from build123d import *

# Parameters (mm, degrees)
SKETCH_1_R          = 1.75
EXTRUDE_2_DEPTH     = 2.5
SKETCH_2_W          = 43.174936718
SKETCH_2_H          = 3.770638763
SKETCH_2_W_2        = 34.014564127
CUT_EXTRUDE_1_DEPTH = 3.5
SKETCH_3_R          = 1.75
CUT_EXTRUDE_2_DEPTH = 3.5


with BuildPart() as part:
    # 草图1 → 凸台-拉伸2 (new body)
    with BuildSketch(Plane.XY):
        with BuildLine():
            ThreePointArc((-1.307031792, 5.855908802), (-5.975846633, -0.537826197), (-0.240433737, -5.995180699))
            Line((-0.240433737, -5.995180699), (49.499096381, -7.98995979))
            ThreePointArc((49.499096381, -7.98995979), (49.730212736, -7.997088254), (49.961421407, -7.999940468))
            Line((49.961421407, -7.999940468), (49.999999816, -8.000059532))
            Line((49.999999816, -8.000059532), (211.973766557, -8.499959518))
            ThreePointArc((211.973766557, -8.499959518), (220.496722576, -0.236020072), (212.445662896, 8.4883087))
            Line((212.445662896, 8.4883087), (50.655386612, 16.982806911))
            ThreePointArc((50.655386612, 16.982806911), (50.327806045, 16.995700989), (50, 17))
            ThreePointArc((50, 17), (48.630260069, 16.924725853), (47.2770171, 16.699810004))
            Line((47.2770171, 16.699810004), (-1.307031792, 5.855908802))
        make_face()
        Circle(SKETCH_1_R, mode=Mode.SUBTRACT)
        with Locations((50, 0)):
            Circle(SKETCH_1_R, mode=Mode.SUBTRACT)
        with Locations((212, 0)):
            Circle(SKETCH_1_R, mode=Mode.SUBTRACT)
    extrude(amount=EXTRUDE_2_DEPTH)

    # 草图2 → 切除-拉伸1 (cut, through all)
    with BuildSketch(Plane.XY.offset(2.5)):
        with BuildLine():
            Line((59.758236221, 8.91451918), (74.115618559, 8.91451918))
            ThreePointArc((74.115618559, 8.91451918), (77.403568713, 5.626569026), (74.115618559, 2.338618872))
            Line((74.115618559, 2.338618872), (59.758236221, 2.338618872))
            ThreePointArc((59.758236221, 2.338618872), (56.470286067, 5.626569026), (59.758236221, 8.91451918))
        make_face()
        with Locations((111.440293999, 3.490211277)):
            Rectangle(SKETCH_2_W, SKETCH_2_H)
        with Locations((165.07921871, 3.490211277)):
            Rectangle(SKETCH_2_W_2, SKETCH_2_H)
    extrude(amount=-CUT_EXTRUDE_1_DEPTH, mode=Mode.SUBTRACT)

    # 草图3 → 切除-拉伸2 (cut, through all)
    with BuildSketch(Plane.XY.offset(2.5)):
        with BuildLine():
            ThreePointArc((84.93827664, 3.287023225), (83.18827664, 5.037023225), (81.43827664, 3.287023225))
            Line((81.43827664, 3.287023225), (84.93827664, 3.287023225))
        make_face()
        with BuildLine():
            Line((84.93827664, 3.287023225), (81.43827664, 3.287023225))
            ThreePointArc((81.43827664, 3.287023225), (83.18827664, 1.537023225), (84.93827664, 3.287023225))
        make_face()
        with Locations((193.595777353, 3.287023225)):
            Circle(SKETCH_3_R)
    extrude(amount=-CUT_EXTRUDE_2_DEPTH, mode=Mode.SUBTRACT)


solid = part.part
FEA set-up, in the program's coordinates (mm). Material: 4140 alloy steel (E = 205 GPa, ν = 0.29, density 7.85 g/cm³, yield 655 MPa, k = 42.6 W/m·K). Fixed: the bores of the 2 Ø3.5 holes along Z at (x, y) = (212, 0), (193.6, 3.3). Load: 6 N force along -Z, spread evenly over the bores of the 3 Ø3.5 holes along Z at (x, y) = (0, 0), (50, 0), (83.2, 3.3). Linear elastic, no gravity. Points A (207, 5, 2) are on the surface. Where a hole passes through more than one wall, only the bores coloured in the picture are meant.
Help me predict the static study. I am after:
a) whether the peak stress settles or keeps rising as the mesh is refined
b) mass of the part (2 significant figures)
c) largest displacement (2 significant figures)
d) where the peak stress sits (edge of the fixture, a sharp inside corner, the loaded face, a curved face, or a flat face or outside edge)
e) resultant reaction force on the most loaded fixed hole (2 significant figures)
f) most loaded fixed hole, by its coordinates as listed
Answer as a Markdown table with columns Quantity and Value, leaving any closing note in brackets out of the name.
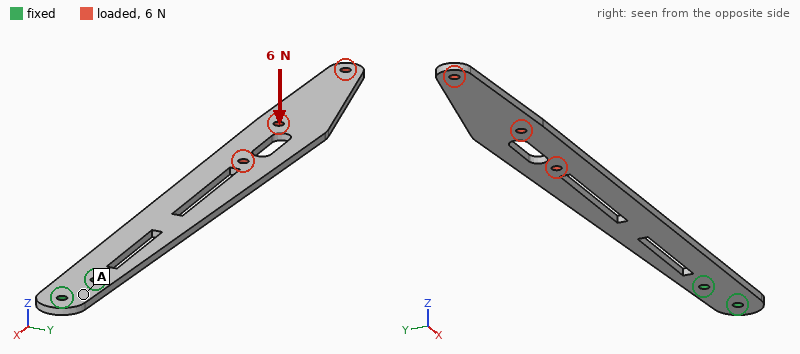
| Quantity | Value |
|---|---|
| whether the peak stress settles or keeps rising as the mesh is refined | keeps rising |
| mass of the part | 79 g |
| largest displacement | 2.2 mm |
| where the peak stress sits | edge of the fixture |
| resultant reaction force on the most loaded fixed hole | 18 N |
| most loaded fixed hole, by its coordinates as listed | (193.6, 3.3) |
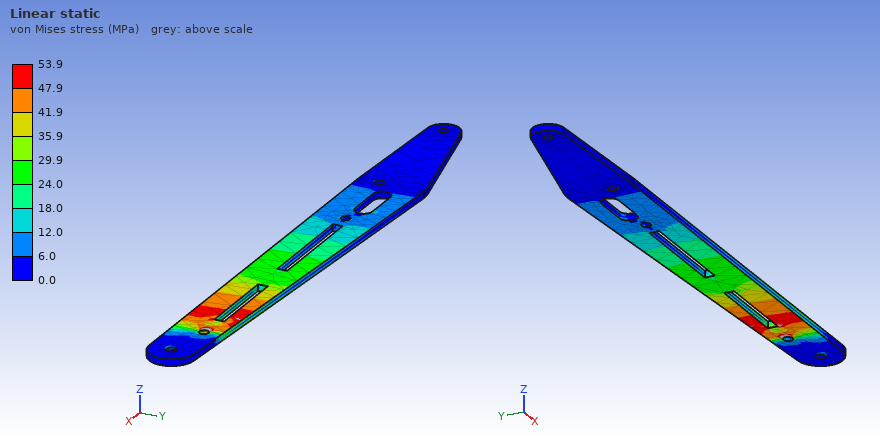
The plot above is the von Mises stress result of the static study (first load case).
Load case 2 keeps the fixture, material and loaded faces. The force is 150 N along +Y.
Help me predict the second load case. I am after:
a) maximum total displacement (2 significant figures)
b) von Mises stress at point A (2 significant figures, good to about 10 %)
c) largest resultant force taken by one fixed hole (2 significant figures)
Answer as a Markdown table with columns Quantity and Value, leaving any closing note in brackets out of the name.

| Quantity | Value |
|---|---|
| maximum total displacement | 0.99 mm |
| von Mises stress at point A | 29 MPa |
| largest resultant force taken by one fixed hole | 1.2 kN |
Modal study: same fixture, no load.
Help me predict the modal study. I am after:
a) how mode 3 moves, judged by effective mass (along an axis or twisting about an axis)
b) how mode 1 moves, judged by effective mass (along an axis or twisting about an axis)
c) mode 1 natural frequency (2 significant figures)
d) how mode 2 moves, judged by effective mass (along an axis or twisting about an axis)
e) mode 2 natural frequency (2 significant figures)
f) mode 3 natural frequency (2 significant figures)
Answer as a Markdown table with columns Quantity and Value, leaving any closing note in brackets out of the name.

| Quantity | Value |
|---|---|
| how mode 3 moves, judged by effective mass | along Y |
| how mode 1 moves, judged by effective mass | along Z |
| mode 1 natural frequency | 52 Hz |
| how mode 2 moves, judged by effective mass | along Z |
| mode 2 natural frequency | 340 Hz |
| mode 3 natural frequency | 370 Hz |
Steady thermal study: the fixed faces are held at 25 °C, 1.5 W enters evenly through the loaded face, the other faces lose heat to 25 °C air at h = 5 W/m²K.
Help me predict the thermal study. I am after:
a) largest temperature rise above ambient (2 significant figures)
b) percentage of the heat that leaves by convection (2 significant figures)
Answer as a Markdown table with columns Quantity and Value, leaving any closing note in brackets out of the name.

| Quantity | Value |
|---|---|
| largest temperature rise above ambient | 46 K |
| percentage of the heat that leaves by convection | 73 % |
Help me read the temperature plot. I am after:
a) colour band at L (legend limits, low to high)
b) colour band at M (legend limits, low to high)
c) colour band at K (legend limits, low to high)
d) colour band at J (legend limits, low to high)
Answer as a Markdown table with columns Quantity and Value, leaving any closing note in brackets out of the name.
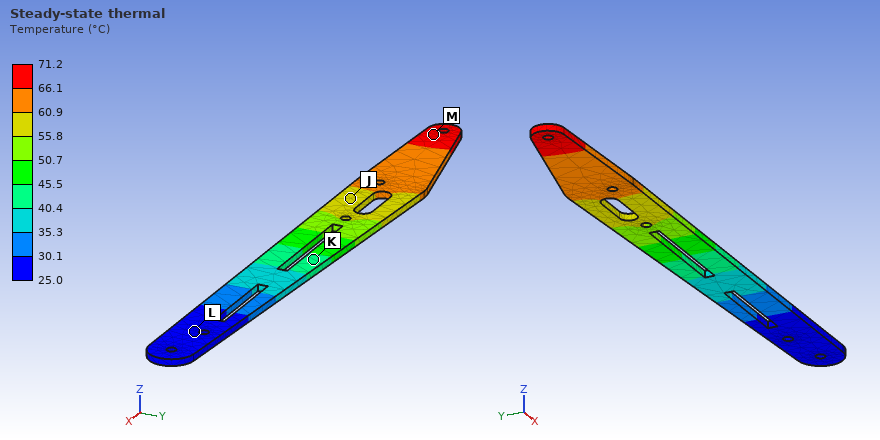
| Quantity | Value |
|---|---|
| colour band at L | 25.0 to 30.1 °C |
| colour band at M | 66.1 to 71.2 °C |
| colour band at K | 40.4 to 45.5 °C |
| colour band at J | 55.8 to 60.9 °C |
